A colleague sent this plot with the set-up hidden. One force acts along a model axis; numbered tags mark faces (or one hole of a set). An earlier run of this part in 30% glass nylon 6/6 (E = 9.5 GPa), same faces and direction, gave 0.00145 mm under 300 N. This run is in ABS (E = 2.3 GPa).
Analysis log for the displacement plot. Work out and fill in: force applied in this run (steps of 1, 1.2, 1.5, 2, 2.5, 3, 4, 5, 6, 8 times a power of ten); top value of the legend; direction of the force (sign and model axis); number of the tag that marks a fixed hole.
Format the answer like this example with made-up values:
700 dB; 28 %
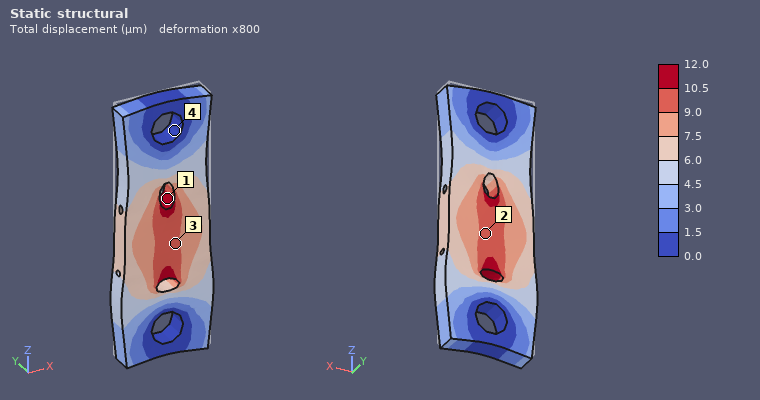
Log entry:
600 N; 12.0 µm; -Z; 4
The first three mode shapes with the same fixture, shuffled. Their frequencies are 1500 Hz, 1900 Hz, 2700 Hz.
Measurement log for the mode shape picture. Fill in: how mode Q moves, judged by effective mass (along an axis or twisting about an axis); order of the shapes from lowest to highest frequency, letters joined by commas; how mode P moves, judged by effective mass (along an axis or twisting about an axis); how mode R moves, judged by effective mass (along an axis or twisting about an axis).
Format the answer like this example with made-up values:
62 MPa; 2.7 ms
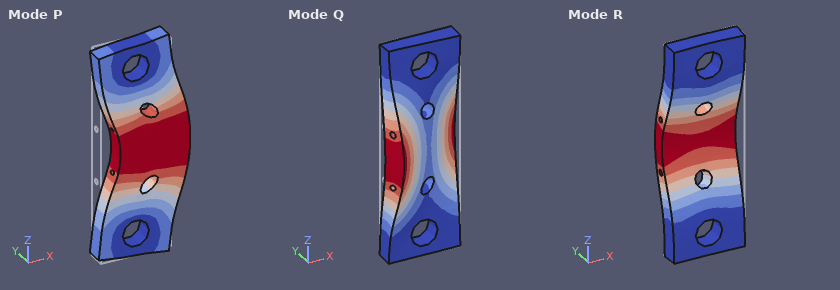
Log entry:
twisting about Z; R, Q, P; along X; along Y
